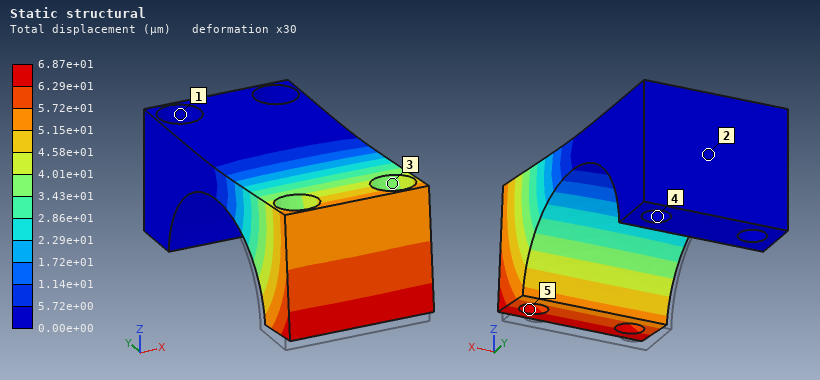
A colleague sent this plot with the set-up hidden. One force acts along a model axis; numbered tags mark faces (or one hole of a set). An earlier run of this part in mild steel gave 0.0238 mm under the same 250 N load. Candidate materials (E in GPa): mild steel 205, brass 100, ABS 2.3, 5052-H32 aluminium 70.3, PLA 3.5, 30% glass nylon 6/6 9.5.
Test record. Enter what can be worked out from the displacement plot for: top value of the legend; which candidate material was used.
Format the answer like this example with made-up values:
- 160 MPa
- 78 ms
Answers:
- 6.87e+01 µm
- 5052-H32 aluminium
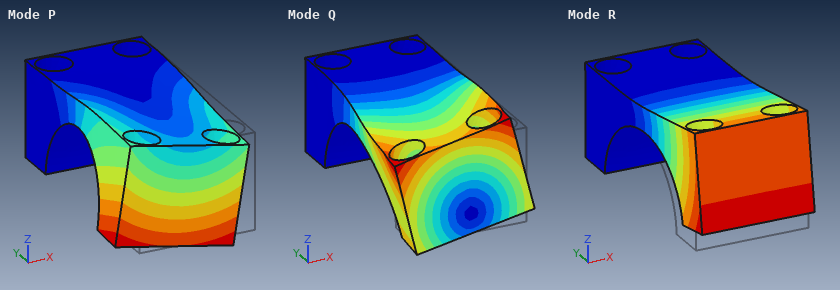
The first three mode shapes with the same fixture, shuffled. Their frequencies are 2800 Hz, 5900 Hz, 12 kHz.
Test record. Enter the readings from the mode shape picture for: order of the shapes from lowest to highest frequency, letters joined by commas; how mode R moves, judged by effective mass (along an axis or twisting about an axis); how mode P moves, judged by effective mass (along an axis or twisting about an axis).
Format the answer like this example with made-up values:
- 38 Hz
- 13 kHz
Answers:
- R, P, Q
- along Z
- along X
